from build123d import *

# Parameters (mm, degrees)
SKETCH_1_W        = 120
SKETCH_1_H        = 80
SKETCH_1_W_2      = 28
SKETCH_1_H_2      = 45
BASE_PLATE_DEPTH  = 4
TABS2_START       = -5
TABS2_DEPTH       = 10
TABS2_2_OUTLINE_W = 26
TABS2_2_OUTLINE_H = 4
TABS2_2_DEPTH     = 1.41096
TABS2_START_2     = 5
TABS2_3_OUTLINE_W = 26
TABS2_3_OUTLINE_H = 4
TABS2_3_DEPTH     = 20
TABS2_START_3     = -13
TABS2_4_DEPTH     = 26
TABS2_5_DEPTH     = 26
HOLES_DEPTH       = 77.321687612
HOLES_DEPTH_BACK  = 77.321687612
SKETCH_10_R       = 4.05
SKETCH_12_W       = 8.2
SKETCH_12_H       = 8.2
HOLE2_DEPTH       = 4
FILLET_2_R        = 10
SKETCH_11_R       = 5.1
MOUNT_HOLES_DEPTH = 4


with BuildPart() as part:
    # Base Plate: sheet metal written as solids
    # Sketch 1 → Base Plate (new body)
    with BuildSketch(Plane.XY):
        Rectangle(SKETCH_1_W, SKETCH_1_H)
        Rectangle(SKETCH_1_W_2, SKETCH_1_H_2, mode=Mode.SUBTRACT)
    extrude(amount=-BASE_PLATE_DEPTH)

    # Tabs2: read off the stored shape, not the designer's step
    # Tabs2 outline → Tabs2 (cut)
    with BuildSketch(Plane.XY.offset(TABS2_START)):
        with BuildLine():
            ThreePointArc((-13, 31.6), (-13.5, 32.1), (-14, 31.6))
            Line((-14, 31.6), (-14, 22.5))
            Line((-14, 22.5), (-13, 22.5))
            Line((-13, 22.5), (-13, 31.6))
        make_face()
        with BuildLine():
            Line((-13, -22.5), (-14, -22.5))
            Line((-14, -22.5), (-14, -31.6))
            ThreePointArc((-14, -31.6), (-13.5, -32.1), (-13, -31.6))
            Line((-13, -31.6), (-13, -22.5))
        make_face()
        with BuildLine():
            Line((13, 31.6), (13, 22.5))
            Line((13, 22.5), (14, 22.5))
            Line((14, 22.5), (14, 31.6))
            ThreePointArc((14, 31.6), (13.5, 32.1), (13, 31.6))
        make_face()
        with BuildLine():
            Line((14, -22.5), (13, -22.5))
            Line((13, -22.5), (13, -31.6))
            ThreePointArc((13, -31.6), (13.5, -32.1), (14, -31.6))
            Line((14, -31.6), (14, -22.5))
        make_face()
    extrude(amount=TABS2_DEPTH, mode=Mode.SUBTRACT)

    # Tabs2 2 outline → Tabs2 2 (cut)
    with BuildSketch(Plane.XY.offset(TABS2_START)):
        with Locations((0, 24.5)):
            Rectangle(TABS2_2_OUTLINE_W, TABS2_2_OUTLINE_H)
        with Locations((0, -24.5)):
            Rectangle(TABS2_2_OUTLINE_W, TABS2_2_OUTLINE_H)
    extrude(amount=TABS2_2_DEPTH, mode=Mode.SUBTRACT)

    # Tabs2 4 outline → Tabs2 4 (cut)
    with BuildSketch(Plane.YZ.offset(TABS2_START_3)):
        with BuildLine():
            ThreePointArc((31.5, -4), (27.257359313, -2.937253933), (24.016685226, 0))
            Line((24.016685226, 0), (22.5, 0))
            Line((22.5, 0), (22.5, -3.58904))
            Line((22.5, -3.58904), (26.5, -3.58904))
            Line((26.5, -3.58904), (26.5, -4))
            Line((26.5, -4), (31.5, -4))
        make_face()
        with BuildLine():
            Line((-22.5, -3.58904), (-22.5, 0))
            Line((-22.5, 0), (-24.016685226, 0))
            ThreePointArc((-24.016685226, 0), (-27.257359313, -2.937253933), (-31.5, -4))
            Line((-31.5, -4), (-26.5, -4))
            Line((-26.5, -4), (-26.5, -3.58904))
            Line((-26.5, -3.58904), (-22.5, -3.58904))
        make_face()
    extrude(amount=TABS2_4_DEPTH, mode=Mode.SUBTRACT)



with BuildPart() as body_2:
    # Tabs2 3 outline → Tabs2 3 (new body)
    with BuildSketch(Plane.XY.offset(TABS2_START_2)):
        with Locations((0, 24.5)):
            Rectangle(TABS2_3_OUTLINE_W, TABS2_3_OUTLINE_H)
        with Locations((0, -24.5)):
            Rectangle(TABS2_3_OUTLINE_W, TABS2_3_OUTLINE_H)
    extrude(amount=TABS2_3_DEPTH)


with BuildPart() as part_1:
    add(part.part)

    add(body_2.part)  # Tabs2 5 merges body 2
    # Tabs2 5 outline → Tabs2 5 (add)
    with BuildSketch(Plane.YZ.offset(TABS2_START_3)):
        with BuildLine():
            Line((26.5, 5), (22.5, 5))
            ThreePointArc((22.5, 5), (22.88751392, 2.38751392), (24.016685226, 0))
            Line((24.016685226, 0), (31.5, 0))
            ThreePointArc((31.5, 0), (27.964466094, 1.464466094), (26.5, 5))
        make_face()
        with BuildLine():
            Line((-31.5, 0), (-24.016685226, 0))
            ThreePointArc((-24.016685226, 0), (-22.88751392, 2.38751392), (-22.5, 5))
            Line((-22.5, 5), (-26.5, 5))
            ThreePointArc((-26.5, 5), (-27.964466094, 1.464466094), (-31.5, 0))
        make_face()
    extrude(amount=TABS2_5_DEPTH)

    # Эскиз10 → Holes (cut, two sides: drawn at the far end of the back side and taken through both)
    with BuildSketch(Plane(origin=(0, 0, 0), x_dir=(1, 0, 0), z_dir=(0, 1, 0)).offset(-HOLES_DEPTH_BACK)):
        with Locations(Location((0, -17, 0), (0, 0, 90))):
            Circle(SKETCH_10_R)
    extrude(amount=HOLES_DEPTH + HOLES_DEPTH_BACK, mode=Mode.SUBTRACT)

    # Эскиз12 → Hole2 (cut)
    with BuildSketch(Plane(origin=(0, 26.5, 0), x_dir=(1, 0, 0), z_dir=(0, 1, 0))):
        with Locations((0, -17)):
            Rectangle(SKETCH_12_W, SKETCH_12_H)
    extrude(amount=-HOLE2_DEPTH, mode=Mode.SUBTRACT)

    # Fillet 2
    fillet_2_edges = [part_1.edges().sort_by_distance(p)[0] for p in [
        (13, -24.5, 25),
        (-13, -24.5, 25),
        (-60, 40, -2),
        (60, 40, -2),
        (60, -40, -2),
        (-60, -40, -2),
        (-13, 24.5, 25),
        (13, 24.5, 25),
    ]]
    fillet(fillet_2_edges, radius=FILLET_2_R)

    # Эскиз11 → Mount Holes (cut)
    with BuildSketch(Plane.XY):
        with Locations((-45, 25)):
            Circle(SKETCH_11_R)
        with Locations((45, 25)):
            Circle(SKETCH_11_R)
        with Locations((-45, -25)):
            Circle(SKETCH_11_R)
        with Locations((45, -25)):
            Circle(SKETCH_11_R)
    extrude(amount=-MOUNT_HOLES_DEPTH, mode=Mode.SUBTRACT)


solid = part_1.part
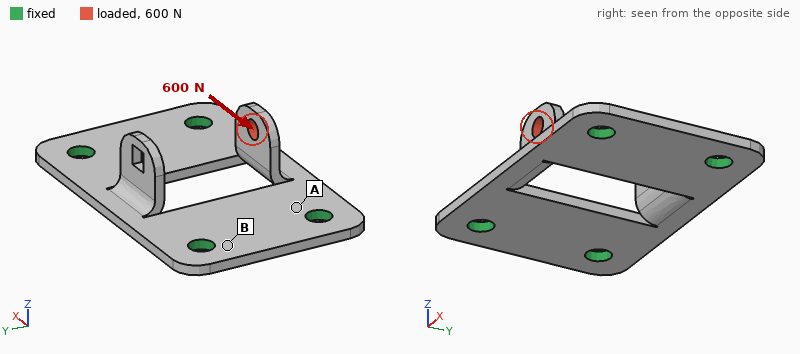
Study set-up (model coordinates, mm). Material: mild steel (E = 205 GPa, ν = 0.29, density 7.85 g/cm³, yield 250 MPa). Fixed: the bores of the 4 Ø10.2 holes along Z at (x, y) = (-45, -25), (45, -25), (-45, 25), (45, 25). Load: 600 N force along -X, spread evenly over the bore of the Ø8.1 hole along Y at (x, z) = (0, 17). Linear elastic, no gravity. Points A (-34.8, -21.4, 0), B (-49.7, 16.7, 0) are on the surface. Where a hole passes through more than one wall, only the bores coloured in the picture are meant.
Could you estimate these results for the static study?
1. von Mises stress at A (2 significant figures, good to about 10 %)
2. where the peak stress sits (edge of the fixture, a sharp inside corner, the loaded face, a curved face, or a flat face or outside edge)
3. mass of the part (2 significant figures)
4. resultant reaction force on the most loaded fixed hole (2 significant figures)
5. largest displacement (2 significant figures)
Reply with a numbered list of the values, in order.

1. 27 MPa
2. a curved face
3. 280 g
4. 490 N
5. 86 µm
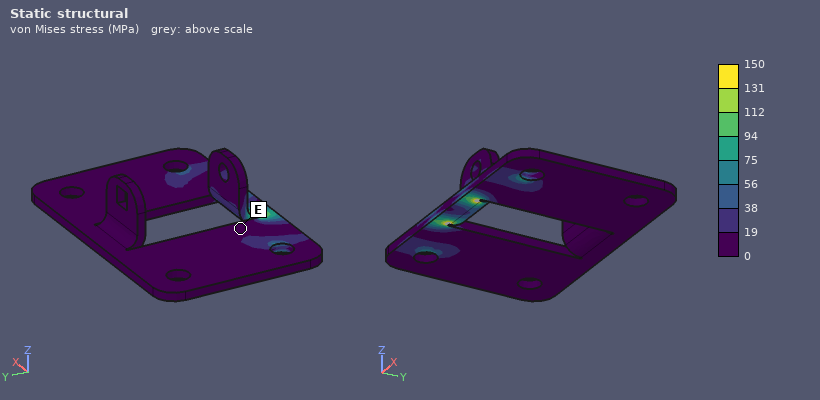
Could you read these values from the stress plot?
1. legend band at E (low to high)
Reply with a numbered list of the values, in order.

1. 0 to 19 MPa
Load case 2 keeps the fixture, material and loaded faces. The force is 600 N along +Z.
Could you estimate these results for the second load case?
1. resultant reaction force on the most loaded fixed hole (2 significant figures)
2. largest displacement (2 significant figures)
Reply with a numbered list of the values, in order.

1. 300 N
2. 0.14 mm
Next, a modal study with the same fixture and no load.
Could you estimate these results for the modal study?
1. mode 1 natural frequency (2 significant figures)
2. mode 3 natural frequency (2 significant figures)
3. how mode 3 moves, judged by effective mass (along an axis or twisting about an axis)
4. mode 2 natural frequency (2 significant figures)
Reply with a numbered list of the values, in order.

1. 2100 Hz
2. 2700 Hz
3. along Z
4. 2200 Hz
